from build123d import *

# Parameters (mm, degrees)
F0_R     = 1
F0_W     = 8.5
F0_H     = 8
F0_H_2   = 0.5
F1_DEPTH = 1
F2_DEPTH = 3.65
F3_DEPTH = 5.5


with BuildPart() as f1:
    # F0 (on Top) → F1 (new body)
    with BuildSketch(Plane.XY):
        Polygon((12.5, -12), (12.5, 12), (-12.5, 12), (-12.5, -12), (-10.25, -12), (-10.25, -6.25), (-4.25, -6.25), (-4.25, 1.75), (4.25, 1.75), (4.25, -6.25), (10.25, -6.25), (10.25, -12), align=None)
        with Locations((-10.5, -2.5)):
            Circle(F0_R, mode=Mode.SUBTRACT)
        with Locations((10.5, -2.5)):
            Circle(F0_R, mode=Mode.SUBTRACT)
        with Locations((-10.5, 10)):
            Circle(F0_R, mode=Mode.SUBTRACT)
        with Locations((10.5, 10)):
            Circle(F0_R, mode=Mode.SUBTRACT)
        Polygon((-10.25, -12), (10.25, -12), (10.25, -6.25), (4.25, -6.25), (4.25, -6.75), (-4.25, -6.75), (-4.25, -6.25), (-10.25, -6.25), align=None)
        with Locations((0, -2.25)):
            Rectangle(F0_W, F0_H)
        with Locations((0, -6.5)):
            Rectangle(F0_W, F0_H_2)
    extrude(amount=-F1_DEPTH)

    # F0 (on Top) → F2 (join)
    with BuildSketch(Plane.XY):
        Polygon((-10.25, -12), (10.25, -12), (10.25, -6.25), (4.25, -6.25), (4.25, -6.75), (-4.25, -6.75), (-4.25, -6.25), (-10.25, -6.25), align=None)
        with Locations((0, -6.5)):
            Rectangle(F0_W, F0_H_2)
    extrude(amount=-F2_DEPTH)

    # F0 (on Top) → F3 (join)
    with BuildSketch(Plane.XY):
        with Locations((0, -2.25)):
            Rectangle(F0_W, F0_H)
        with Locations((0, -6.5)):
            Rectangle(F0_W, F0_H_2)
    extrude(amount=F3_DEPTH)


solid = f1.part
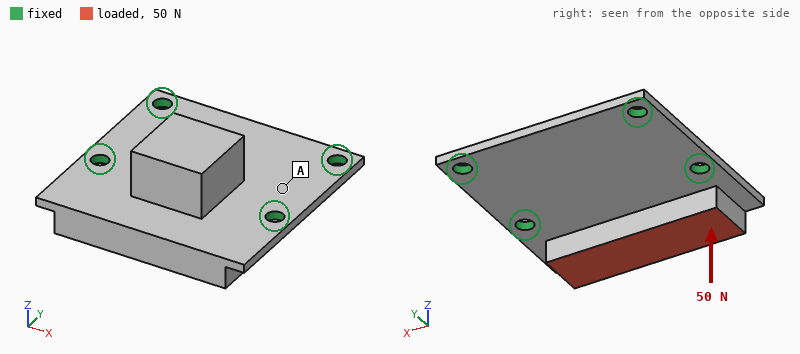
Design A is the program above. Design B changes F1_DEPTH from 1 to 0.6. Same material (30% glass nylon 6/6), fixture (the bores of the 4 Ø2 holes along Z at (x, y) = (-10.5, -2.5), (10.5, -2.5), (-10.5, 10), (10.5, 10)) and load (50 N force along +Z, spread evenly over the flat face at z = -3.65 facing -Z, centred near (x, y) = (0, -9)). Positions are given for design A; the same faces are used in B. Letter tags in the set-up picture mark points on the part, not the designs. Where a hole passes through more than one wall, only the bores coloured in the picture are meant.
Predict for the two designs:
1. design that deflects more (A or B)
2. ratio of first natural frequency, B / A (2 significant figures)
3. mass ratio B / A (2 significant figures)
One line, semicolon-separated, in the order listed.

B; 0.56; 0.86
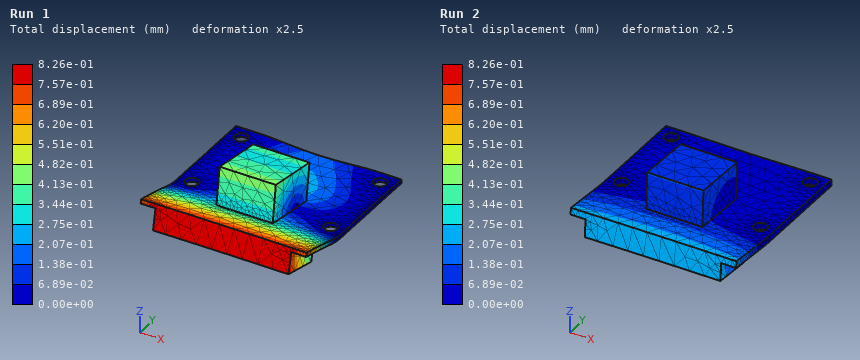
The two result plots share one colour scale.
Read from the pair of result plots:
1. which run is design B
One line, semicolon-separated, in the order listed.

Run 1
